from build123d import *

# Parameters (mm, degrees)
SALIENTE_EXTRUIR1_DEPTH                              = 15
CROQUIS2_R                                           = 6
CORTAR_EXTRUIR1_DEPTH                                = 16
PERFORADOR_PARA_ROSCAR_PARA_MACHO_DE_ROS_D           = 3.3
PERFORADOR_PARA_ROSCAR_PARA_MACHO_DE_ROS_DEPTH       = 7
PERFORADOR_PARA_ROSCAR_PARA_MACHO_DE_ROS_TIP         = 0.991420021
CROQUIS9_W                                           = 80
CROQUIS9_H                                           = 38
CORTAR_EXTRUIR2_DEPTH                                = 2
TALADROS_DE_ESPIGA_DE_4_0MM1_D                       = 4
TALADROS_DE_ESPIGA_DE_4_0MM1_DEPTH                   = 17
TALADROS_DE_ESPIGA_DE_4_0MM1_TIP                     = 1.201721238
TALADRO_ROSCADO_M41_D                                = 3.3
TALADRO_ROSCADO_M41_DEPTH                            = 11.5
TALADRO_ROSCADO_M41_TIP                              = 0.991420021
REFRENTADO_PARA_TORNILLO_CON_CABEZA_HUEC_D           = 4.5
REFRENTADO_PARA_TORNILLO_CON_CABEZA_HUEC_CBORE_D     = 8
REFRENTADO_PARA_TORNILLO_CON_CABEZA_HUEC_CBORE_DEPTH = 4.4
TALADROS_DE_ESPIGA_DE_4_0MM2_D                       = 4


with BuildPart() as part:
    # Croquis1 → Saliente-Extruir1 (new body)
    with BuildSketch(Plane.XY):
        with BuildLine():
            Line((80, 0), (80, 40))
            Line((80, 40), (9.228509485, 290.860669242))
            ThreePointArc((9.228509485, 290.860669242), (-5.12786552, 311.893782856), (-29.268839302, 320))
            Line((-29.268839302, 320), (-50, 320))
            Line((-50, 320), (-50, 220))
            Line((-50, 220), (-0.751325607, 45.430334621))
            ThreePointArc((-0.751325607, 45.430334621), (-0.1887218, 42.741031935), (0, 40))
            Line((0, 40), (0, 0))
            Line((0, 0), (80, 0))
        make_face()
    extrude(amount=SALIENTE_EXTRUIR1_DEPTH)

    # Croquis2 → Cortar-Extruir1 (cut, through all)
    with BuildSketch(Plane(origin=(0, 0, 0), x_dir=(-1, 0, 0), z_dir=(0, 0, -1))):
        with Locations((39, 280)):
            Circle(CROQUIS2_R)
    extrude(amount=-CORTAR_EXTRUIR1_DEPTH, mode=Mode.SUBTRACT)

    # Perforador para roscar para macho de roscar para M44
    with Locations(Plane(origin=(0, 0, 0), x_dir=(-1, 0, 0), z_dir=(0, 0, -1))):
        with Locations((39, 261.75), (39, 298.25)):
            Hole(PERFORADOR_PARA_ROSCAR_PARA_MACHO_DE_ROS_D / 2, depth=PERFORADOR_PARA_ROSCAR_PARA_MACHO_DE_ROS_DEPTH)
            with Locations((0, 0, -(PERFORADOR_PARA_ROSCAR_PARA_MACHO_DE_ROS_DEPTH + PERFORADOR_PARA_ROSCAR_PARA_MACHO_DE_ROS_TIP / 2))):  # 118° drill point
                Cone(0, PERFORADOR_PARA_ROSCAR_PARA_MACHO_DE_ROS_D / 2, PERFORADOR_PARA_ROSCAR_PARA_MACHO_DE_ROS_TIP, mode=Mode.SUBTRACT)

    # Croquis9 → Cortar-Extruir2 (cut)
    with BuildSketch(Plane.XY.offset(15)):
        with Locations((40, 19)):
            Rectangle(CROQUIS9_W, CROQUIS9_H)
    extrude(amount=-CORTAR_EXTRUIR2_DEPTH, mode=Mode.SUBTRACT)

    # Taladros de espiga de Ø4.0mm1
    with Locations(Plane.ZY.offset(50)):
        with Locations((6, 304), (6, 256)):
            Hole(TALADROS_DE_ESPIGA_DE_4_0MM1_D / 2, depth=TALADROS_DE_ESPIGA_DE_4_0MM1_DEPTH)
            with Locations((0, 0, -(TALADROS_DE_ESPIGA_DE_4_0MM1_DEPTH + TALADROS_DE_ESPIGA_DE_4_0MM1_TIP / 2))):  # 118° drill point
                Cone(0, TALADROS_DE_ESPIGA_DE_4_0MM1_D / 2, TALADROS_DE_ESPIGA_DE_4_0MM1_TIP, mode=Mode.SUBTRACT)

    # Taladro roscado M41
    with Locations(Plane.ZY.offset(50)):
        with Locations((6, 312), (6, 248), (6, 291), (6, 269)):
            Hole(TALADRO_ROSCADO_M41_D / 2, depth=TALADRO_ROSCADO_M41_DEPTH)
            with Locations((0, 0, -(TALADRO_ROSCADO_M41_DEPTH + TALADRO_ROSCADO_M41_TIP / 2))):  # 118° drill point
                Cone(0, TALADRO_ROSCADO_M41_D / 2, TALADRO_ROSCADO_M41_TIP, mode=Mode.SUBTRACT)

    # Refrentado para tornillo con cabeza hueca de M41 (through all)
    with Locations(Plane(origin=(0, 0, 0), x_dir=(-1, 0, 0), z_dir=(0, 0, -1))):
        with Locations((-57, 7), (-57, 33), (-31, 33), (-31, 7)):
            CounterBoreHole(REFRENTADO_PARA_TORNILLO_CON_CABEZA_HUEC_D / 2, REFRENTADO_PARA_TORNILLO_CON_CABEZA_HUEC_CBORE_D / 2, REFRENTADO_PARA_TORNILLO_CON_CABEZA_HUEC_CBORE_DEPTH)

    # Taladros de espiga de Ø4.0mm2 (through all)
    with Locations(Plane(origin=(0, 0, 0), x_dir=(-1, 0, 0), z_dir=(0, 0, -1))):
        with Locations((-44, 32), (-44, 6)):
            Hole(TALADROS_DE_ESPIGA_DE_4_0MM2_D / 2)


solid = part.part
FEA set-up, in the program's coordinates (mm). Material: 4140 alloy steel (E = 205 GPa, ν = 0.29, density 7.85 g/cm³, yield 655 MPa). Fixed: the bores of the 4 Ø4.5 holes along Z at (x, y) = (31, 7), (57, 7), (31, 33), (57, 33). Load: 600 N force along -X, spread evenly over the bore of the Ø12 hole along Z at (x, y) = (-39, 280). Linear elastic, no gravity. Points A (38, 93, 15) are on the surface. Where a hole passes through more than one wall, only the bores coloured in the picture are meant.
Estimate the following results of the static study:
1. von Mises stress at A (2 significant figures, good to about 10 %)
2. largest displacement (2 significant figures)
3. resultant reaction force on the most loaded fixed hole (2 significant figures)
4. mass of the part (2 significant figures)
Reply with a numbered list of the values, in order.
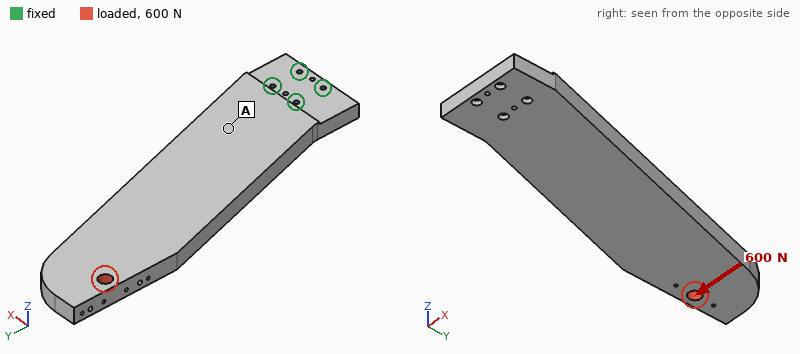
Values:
1. 2.8 MPa
2. 53 µm
3. 2.8 kN
4. 2.7 kg
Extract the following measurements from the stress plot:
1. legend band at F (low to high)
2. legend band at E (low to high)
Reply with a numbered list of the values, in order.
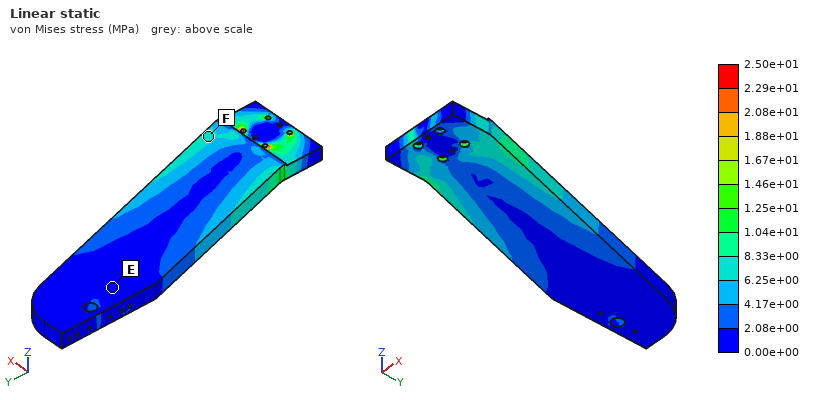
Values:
1. 6.25e+00 to 8.33e+00 MPa
2. 0.00e+00 to 2.08e+00 MPa
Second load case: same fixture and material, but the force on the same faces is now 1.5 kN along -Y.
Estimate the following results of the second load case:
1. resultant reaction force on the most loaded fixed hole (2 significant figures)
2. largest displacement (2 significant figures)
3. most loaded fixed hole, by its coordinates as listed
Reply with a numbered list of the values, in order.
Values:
1. 2.6 kN
2. 47 µm
3. (31, 33)
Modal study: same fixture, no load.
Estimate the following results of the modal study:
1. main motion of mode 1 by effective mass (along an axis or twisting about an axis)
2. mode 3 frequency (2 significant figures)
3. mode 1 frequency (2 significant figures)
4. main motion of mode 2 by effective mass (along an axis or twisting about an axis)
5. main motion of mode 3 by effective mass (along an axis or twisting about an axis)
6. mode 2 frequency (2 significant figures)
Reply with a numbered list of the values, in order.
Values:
1. along Z
2. 870 Hz
3. 150 Hz
4. along X
5. along Z
6. 630 Hz
